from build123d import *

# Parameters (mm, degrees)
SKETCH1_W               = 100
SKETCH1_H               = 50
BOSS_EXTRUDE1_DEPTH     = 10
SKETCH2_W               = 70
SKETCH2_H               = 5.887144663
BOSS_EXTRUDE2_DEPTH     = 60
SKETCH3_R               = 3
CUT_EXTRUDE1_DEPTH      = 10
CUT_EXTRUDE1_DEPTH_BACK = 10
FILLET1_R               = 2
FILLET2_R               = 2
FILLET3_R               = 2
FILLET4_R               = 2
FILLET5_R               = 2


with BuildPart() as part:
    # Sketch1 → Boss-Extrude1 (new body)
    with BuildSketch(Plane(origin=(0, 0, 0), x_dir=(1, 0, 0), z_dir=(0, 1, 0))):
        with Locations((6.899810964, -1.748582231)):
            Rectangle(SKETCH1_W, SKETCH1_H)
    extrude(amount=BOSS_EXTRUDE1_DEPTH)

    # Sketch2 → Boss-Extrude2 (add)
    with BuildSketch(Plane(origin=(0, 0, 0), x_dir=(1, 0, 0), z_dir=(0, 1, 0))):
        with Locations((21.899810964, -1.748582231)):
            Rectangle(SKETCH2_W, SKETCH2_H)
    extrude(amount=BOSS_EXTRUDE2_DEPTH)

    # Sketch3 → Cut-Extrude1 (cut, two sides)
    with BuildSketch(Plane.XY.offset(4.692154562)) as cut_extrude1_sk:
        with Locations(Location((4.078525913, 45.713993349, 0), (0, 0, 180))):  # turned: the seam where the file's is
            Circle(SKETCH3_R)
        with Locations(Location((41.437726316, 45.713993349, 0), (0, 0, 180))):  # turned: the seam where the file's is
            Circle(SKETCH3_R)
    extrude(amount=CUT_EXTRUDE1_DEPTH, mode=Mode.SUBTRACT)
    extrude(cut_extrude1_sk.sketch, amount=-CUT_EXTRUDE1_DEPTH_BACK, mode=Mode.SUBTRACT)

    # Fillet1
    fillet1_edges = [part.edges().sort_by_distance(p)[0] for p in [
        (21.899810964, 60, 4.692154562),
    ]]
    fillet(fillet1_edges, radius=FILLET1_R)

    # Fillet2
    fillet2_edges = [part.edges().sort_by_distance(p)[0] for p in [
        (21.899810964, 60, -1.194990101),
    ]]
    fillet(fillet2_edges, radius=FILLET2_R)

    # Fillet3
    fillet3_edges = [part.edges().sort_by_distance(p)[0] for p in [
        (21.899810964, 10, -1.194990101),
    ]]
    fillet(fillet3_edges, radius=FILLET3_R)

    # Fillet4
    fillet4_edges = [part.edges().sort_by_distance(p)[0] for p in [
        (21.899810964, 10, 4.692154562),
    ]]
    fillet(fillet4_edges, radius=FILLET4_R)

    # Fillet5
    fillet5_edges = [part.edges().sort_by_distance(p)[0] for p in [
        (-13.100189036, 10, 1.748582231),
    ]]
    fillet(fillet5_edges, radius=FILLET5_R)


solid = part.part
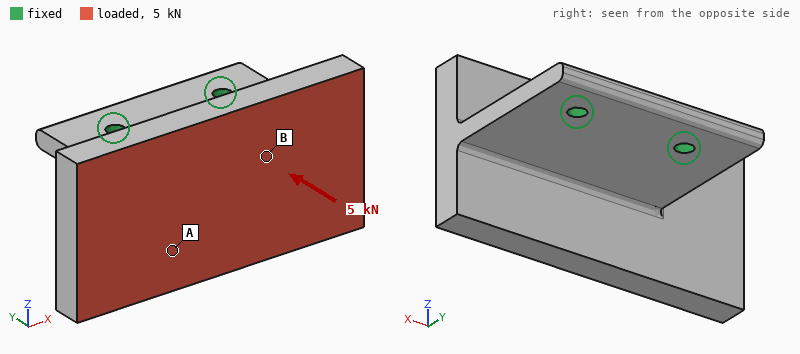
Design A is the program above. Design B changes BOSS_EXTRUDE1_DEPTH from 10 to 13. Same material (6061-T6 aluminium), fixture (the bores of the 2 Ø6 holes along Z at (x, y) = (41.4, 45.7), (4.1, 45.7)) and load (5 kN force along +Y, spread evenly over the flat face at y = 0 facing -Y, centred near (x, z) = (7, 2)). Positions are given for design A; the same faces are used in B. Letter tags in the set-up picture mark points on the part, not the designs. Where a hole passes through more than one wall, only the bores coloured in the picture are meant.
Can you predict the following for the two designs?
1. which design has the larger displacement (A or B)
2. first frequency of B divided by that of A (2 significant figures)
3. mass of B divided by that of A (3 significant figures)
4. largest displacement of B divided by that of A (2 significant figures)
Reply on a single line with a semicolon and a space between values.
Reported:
A; 0.93; 1.20; 0.69
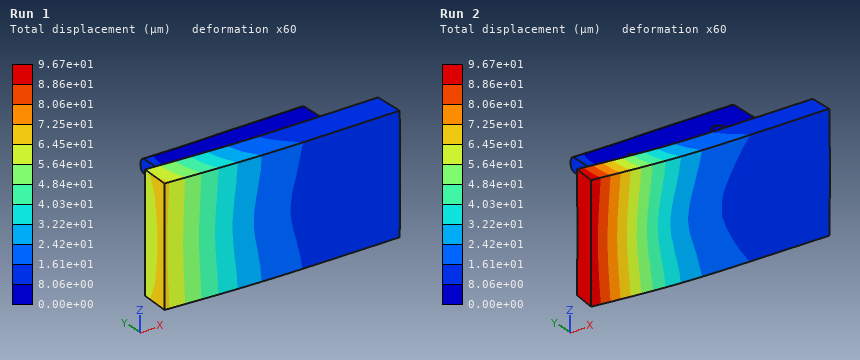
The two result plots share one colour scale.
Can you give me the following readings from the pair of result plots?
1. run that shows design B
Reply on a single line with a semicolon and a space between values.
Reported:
Run 1
